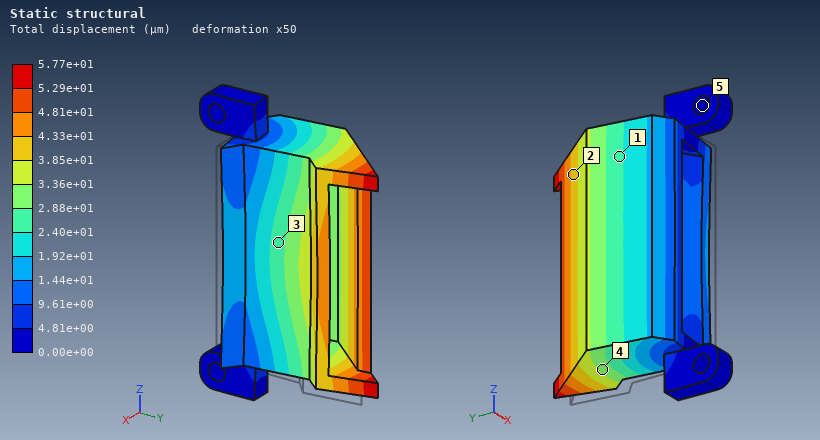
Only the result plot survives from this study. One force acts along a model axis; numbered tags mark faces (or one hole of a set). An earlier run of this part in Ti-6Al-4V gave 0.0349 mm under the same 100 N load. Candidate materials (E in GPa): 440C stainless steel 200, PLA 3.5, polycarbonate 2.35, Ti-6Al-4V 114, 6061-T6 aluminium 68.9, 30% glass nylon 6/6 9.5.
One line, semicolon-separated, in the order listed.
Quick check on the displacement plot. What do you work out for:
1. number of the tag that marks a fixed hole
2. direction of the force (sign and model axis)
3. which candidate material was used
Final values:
5; -X; 6061-T6 aluminium
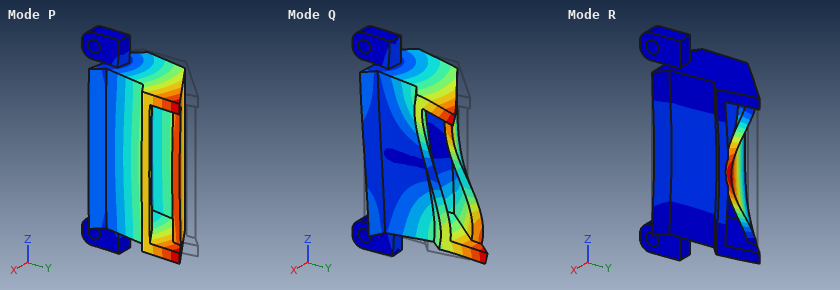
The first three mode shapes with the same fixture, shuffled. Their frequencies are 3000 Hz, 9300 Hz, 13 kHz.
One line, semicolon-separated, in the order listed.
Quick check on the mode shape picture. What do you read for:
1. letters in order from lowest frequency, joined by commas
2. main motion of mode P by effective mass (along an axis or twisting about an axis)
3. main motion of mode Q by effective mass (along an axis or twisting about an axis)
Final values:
P, Q, R; along X; twisting about Y
